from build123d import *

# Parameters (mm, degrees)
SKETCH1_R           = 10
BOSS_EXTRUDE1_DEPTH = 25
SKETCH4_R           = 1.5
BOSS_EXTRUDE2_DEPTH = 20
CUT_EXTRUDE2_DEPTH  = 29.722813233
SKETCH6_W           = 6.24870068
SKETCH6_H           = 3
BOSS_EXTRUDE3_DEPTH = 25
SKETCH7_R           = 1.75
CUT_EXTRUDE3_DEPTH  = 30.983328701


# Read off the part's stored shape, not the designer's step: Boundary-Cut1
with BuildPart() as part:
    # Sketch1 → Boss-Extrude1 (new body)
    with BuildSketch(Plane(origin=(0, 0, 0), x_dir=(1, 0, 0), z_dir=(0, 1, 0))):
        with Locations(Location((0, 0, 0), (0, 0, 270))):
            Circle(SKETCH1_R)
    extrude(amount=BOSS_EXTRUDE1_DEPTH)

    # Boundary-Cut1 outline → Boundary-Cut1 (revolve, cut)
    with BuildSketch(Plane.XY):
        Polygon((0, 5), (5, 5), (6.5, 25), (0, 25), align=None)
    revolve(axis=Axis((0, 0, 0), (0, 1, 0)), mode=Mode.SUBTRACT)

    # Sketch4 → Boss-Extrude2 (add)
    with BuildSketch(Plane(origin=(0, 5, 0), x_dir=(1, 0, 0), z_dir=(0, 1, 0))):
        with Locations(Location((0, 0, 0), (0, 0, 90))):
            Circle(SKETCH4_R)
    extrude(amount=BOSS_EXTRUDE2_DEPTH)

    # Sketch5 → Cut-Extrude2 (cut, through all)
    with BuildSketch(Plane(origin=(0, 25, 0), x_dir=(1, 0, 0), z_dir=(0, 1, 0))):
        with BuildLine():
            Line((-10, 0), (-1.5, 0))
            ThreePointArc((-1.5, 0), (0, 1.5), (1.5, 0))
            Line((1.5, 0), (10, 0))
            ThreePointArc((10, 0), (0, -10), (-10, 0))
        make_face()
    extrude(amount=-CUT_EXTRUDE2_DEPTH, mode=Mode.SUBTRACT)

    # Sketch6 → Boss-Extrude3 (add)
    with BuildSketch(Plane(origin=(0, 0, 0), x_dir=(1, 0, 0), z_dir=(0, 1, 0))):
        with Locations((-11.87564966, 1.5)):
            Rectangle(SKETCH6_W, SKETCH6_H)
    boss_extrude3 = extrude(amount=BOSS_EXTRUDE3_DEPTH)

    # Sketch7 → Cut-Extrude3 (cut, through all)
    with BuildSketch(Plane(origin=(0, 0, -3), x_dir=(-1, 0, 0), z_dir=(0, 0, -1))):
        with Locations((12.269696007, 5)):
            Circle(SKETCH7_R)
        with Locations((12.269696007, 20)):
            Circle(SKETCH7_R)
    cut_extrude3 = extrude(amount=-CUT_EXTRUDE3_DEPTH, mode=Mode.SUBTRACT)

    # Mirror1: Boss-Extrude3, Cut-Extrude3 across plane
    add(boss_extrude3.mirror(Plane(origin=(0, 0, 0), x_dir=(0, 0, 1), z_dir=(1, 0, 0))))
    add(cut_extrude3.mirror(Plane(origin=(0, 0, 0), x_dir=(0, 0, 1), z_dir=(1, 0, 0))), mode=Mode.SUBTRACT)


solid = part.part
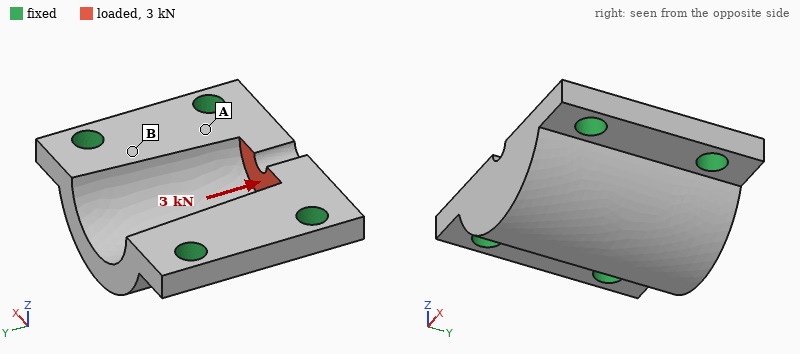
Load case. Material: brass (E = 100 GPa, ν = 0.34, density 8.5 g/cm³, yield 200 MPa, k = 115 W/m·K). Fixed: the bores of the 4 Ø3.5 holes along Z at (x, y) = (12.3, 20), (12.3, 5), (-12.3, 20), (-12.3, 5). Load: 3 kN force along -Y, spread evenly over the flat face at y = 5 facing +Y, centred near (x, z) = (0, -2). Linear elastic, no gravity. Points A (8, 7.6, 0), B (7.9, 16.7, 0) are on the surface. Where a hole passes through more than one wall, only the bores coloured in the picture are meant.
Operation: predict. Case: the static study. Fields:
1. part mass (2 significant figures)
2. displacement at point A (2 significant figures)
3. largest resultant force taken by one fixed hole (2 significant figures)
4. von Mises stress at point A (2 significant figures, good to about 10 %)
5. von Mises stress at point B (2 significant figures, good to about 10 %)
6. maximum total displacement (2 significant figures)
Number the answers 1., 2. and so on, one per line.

1. 30 g
2. 3.6 µm
3. 880 N
4. 54 MPa
5. 24 MPa
6. 18 µm
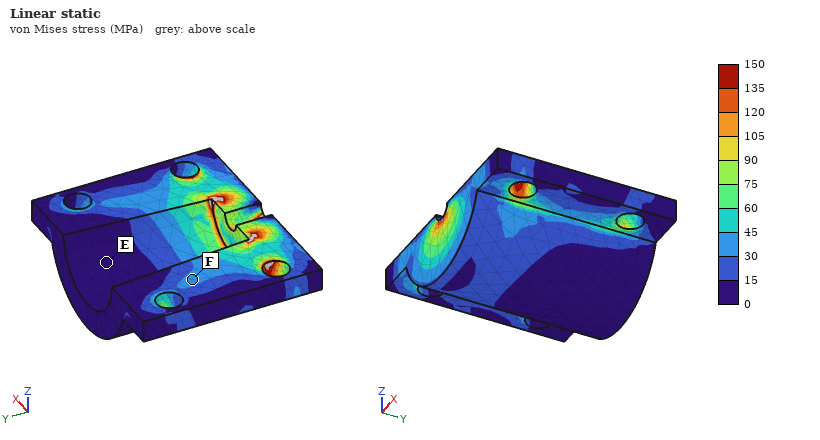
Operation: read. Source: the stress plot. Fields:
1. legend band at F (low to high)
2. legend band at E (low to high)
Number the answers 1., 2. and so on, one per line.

1. 30 to 45 MPa
2. 0 to 15 MPa
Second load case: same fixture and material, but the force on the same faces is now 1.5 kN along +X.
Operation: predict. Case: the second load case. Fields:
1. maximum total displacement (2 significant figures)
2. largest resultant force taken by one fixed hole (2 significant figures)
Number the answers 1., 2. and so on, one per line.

1. 5.3 µm
2. 680 N
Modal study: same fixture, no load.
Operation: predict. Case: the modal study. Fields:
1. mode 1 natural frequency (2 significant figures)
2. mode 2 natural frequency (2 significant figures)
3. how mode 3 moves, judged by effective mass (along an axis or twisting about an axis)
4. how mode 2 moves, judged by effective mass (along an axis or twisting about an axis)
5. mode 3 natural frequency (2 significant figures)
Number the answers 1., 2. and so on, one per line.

1. 20 kHz
2. 25 kHz
3. along X
4. along Z
5. 33 kHz
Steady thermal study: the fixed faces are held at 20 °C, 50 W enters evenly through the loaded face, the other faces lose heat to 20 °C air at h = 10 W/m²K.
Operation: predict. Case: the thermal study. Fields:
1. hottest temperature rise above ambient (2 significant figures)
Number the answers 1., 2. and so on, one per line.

1. 63 K
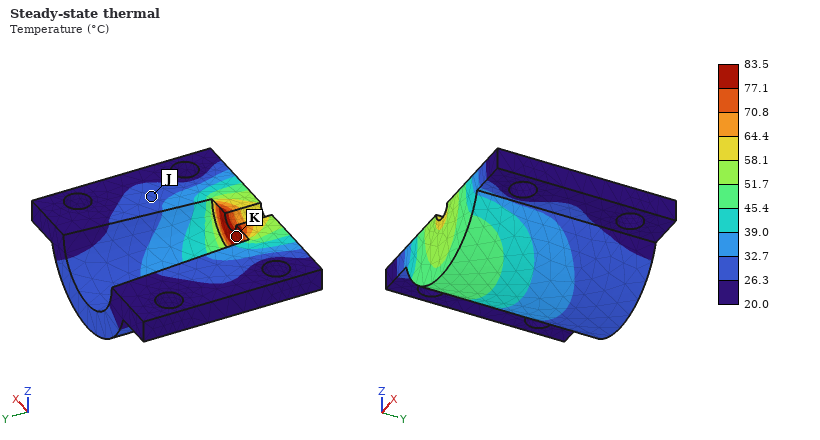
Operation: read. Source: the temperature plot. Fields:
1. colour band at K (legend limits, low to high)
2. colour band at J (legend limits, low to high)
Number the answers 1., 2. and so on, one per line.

1. 77.1 to 83.5 °C
2. 26.3 to 32.7 °C
